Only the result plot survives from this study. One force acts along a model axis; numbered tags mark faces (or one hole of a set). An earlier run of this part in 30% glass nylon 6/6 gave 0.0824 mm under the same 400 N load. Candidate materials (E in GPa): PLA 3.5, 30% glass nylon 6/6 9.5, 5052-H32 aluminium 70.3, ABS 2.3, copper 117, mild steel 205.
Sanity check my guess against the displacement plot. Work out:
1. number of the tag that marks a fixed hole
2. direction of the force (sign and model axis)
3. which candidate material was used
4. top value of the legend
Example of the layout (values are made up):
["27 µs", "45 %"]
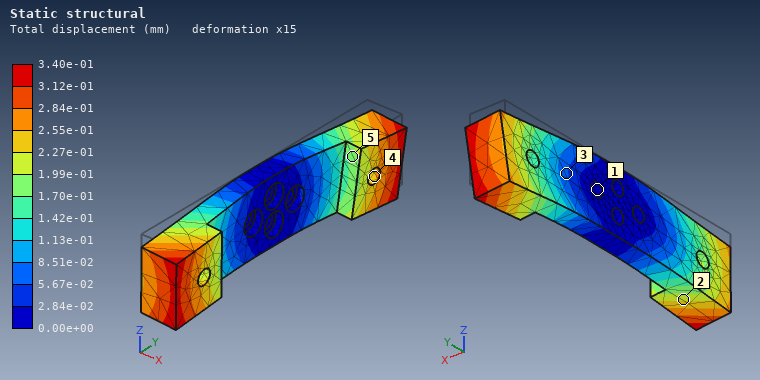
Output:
["1", "-Z", "ABS", "3.40e-01 mm"]
